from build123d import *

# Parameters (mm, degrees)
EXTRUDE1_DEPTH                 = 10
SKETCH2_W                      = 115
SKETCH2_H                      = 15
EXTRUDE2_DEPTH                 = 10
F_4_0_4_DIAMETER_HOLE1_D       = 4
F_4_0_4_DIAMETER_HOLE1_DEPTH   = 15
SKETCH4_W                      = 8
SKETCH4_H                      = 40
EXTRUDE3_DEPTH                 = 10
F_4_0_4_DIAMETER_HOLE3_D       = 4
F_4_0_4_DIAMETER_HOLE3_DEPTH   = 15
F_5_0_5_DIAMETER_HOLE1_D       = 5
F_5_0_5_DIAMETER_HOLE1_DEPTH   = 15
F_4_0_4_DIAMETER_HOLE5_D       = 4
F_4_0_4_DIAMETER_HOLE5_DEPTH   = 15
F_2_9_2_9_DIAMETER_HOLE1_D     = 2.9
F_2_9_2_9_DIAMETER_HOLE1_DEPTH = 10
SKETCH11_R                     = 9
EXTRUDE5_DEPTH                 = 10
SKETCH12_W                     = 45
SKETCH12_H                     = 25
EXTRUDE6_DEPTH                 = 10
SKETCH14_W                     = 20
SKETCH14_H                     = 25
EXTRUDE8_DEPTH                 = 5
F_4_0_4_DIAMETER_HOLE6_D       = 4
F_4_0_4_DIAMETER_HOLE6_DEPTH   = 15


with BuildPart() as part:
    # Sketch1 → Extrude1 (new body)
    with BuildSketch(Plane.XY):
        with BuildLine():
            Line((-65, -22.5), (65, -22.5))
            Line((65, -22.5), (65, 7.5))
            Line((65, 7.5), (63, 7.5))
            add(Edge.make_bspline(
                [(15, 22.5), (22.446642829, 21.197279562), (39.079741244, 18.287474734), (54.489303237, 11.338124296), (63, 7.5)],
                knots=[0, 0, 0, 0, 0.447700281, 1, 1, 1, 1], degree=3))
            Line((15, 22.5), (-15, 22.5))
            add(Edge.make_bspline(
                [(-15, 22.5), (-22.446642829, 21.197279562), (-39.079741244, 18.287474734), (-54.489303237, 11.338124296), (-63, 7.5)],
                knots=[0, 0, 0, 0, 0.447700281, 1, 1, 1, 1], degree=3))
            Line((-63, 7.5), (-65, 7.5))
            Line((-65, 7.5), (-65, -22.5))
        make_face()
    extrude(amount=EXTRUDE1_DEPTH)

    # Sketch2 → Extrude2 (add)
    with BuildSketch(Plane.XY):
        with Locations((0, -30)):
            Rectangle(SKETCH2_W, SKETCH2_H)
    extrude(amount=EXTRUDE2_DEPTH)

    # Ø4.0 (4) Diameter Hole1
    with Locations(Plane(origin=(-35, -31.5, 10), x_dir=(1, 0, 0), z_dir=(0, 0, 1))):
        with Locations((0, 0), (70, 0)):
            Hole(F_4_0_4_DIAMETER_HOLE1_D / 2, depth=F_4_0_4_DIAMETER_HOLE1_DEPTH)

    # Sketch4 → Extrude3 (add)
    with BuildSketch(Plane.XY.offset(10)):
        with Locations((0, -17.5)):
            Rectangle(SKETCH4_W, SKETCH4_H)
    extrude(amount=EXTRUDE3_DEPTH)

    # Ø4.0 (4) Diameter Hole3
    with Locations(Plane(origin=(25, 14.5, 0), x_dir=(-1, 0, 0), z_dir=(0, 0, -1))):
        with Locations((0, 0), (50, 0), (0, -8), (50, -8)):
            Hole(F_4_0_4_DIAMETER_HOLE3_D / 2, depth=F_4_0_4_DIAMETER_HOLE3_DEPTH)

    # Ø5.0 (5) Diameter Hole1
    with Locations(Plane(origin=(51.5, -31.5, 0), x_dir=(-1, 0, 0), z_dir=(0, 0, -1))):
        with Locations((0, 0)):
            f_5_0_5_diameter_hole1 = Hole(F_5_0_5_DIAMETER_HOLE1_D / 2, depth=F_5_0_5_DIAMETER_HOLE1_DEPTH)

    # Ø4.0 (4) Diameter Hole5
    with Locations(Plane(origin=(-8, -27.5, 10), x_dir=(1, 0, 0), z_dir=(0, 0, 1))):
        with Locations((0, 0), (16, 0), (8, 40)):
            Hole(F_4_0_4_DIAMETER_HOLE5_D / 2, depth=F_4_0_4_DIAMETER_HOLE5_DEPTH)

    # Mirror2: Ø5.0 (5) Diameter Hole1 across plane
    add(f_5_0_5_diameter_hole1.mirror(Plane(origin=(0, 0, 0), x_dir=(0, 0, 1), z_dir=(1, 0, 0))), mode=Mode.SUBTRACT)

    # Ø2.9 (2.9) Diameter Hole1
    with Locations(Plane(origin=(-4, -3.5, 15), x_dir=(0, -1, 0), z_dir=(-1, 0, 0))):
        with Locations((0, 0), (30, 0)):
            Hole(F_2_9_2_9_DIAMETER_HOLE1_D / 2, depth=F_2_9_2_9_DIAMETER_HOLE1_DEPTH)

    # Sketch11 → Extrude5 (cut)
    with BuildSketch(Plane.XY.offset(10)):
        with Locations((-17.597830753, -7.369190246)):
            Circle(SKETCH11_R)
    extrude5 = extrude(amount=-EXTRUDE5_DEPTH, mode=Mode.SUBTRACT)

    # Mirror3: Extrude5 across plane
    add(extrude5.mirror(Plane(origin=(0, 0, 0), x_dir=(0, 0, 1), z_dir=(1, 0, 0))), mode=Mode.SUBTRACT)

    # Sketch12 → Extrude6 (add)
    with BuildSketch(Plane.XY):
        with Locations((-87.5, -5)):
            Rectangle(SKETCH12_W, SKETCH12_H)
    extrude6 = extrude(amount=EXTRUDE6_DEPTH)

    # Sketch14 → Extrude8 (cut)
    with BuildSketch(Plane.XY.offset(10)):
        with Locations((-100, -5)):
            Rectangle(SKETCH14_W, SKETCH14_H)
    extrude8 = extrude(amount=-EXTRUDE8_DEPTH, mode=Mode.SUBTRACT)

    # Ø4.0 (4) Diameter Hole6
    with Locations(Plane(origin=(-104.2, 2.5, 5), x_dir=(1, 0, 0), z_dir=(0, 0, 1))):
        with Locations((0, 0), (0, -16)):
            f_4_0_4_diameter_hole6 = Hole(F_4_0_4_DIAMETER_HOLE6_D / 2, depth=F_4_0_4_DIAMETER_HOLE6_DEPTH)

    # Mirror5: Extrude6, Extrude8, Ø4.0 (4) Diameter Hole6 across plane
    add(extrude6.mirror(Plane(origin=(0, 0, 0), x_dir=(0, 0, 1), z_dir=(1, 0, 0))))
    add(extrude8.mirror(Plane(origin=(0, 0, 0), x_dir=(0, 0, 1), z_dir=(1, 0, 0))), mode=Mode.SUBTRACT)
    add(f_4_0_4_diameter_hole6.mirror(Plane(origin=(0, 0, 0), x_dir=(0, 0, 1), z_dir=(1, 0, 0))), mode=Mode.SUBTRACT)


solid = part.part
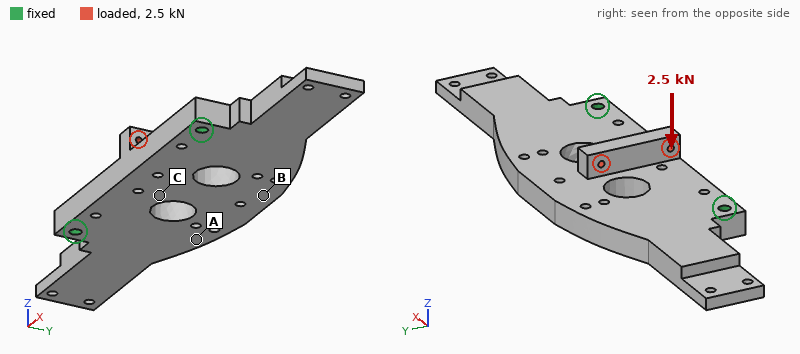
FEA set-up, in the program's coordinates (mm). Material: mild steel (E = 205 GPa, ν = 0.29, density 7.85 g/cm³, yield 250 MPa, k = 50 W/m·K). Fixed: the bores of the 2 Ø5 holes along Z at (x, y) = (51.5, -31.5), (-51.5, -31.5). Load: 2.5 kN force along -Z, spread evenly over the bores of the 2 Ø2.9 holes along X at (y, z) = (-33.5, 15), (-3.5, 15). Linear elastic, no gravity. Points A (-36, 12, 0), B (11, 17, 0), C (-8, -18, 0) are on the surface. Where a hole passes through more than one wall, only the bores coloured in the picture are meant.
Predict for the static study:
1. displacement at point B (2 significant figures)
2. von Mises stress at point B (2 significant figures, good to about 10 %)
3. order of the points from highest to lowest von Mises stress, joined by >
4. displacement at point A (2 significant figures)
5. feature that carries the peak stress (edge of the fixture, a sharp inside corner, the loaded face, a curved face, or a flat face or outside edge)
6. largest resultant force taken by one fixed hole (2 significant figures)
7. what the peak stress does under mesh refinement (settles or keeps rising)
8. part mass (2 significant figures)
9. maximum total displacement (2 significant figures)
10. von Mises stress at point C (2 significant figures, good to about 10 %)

50 µm
24 MPa
C > B > A
33 µm
edge of the fixture
1.3 kN
keeps rising
650 g
55 µm
44 MPa
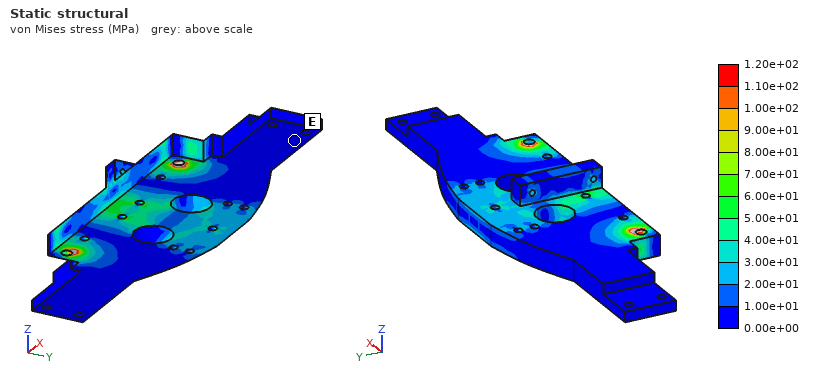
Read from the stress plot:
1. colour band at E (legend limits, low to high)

0.00e+00 to 1.00e+01 MPa
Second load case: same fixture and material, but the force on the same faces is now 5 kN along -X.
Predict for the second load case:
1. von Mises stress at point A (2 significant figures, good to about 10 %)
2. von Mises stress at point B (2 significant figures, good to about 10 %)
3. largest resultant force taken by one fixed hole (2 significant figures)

9.4 MPa
11 MPa
2.6 kN
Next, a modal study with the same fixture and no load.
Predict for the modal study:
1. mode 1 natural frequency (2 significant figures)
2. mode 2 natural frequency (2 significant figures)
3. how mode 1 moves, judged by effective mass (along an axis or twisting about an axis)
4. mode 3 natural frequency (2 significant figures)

1700 Hz
2000 Hz
along Z
2100 Hz
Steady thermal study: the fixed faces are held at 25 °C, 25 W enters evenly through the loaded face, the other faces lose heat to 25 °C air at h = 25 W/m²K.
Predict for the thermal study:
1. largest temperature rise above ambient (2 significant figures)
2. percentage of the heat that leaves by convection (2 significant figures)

54 K
37 %
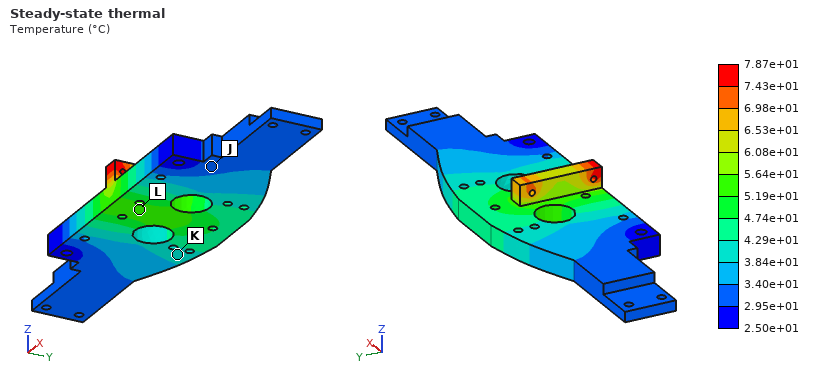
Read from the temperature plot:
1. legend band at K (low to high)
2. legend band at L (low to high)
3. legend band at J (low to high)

3.84e+01 to 4.29e+01 °C
5.19e+01 to 5.64e+01 °C
2.95e+01 to 3.40e+01 °C
